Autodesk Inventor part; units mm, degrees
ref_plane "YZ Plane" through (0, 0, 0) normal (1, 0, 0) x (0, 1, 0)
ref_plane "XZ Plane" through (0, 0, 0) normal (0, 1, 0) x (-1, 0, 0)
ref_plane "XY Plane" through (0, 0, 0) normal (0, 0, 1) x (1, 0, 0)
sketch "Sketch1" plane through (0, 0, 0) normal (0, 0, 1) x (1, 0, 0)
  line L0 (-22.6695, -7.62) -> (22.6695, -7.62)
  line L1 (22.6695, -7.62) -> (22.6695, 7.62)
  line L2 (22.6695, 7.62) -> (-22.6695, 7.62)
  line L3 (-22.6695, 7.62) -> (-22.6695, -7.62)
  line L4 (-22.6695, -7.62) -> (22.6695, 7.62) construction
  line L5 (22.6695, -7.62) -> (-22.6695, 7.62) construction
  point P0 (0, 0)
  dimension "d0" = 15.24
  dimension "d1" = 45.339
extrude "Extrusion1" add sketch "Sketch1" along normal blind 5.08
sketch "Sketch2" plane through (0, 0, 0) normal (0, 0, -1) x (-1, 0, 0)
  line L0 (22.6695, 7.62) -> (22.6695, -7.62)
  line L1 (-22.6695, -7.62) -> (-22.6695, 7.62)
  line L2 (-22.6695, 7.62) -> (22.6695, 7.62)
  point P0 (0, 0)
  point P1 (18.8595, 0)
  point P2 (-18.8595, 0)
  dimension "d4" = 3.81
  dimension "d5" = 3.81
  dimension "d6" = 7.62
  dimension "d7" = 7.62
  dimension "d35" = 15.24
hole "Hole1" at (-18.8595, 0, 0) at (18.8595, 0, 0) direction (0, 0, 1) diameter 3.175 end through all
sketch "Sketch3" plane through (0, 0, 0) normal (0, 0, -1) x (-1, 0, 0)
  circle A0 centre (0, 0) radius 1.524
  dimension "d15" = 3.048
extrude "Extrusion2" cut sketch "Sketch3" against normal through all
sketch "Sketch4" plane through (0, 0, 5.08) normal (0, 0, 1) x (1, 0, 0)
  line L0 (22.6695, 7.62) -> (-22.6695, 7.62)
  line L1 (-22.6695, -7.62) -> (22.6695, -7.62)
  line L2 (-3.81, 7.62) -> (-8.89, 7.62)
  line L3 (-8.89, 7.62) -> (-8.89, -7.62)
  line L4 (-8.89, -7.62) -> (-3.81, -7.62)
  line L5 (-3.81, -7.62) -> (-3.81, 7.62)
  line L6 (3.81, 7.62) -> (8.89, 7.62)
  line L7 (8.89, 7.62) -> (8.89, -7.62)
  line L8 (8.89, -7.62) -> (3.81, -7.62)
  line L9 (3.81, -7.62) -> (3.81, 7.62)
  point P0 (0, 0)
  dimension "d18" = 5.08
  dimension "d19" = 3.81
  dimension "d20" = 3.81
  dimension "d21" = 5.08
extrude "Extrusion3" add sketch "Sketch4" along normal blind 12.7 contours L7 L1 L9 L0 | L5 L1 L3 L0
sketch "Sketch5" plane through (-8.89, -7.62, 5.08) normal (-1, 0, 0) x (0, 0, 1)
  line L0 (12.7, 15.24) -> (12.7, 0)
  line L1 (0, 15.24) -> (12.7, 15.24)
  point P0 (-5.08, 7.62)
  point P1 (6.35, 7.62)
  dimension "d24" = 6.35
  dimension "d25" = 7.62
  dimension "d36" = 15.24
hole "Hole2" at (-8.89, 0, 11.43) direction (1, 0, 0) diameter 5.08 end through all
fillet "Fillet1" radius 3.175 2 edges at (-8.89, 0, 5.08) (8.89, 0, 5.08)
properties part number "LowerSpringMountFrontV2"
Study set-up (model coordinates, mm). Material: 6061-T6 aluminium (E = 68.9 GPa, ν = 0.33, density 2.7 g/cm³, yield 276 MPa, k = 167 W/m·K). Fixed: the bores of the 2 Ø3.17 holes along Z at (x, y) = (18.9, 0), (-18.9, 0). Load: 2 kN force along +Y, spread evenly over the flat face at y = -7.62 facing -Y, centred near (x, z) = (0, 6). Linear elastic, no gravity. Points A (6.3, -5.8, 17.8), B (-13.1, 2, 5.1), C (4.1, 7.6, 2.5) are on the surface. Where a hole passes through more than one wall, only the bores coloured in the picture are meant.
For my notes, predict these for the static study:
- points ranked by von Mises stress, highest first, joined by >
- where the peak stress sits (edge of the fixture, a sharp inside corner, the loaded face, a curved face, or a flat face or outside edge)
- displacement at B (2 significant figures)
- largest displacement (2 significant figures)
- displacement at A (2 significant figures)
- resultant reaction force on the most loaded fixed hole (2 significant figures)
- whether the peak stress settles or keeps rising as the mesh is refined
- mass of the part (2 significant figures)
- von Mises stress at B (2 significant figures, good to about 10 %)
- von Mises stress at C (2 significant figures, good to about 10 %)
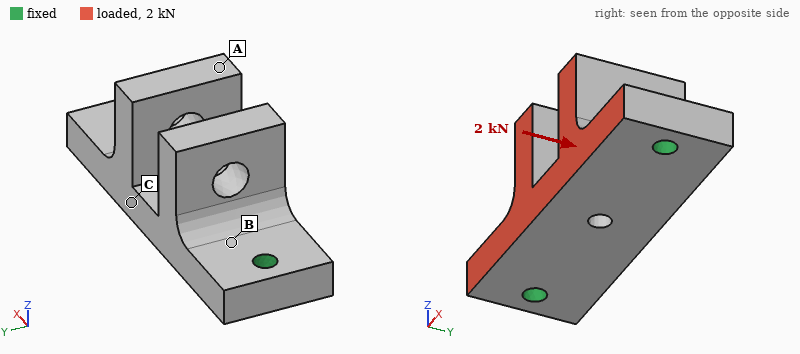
B > C > A
edge of the fixture
9.8 µm
52 µm
50 µm
1.0 kN
keeps rising
14 g
59 MPa
32 MPa
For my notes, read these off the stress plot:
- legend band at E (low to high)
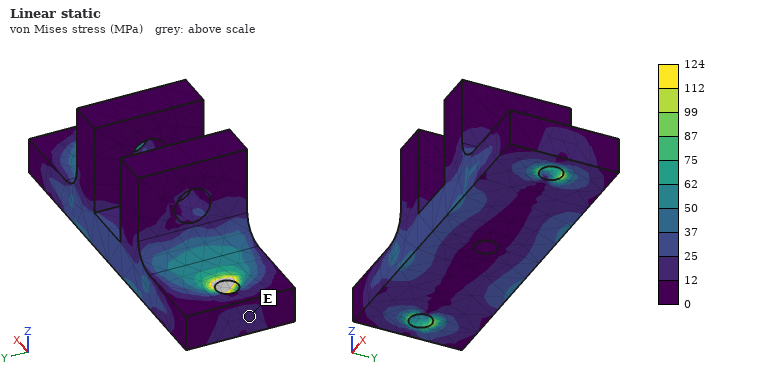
12 to 25 MPa
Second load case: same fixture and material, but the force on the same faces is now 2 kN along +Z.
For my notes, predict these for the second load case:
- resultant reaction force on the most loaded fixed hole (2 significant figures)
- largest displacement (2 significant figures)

1.0 kN
99 µm
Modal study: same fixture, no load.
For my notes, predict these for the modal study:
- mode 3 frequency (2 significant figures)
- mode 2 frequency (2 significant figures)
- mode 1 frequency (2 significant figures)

18 kHz
10000 Hz
9700 Hz
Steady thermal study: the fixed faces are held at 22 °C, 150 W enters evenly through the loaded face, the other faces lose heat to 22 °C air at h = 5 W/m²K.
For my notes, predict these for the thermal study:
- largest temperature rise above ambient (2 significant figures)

84 K
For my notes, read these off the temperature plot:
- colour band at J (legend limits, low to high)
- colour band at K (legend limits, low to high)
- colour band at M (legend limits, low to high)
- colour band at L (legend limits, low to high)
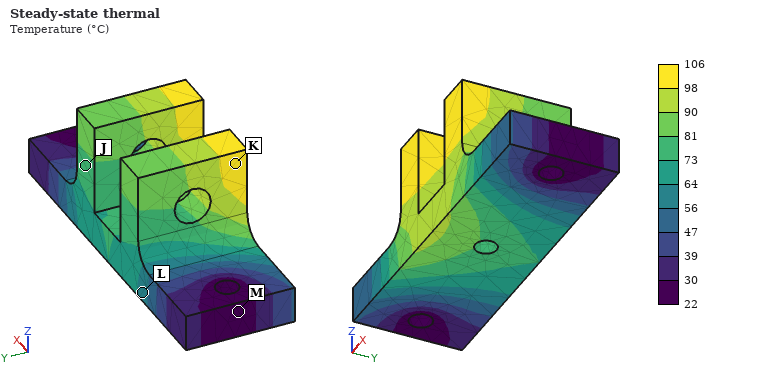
73 to 81 °C
98 to 106 °C
22 to 30 °C
56 to 64 °C
